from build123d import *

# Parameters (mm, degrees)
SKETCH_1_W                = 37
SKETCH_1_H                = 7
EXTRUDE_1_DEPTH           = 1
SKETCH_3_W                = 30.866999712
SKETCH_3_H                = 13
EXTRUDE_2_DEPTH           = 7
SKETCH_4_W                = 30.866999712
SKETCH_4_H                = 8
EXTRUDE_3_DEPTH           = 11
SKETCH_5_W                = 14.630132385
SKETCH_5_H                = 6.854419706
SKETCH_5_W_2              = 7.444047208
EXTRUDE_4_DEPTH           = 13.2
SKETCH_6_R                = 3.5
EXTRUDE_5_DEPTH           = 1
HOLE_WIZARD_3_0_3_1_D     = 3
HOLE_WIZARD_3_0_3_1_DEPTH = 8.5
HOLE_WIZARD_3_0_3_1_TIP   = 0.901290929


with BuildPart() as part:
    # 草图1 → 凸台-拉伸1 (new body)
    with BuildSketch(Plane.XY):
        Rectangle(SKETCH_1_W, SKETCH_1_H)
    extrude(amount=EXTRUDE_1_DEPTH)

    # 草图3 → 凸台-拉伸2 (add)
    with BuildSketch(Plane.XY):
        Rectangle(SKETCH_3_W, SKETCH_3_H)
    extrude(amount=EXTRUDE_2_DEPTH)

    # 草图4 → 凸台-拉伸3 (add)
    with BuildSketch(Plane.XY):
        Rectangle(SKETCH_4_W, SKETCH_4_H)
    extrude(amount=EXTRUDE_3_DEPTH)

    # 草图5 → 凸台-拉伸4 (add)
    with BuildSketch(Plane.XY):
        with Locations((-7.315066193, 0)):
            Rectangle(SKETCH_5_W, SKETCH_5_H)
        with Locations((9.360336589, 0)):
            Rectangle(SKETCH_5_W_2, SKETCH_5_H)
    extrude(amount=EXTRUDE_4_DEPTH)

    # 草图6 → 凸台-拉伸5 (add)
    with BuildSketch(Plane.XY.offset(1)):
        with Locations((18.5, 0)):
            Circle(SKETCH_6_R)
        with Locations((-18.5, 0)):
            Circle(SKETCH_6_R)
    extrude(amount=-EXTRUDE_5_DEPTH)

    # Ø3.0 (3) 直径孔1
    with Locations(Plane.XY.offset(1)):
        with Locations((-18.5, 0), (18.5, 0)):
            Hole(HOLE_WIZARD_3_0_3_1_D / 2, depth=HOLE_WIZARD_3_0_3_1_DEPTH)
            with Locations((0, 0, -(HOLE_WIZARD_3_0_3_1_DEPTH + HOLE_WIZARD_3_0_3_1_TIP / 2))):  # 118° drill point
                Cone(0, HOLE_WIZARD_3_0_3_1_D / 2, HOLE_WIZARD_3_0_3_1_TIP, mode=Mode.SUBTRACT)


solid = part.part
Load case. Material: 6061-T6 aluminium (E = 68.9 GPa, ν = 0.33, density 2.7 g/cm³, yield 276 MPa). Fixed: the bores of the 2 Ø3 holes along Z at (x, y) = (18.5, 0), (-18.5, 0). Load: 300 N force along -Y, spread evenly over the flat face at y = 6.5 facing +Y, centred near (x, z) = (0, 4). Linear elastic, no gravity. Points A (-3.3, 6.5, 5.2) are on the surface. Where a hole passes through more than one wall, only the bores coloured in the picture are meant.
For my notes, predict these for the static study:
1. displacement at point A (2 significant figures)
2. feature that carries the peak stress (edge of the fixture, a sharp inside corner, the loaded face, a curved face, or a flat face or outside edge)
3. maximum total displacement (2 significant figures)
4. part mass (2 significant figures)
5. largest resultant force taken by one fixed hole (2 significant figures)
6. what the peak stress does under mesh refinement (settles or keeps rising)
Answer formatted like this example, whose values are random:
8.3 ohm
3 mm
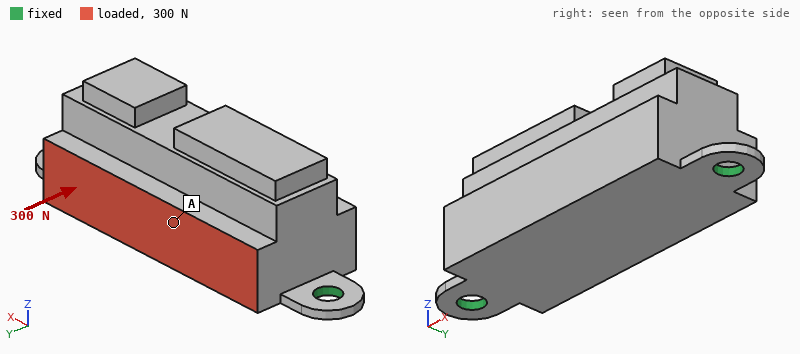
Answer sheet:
0.066 mm
edge of the fixture
0.11 mm
11 g
150 N
keeps rising
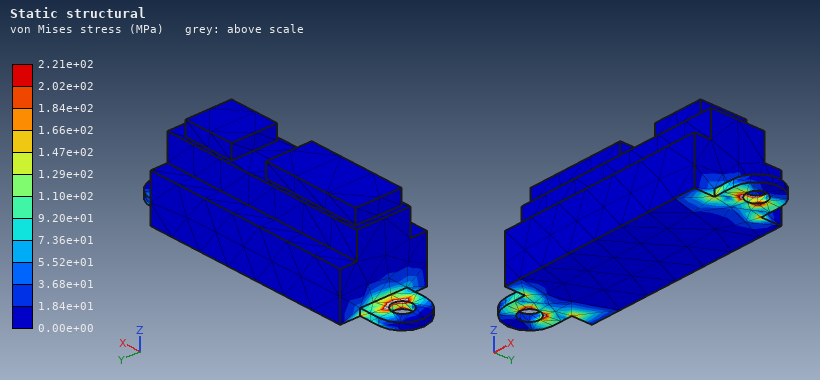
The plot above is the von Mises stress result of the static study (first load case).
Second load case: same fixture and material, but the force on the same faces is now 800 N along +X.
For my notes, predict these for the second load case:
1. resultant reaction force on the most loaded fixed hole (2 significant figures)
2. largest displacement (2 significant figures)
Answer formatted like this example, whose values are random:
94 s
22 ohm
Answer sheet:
430 N
8.3 µm
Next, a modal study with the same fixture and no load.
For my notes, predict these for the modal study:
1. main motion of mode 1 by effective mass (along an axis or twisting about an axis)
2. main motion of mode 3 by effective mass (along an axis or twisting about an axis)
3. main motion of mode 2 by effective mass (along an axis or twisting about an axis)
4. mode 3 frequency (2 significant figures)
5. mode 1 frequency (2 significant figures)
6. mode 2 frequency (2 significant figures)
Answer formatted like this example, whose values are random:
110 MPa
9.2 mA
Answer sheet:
along Y
along X
along Z
14 kHz
2300 Hz
9000 Hz
